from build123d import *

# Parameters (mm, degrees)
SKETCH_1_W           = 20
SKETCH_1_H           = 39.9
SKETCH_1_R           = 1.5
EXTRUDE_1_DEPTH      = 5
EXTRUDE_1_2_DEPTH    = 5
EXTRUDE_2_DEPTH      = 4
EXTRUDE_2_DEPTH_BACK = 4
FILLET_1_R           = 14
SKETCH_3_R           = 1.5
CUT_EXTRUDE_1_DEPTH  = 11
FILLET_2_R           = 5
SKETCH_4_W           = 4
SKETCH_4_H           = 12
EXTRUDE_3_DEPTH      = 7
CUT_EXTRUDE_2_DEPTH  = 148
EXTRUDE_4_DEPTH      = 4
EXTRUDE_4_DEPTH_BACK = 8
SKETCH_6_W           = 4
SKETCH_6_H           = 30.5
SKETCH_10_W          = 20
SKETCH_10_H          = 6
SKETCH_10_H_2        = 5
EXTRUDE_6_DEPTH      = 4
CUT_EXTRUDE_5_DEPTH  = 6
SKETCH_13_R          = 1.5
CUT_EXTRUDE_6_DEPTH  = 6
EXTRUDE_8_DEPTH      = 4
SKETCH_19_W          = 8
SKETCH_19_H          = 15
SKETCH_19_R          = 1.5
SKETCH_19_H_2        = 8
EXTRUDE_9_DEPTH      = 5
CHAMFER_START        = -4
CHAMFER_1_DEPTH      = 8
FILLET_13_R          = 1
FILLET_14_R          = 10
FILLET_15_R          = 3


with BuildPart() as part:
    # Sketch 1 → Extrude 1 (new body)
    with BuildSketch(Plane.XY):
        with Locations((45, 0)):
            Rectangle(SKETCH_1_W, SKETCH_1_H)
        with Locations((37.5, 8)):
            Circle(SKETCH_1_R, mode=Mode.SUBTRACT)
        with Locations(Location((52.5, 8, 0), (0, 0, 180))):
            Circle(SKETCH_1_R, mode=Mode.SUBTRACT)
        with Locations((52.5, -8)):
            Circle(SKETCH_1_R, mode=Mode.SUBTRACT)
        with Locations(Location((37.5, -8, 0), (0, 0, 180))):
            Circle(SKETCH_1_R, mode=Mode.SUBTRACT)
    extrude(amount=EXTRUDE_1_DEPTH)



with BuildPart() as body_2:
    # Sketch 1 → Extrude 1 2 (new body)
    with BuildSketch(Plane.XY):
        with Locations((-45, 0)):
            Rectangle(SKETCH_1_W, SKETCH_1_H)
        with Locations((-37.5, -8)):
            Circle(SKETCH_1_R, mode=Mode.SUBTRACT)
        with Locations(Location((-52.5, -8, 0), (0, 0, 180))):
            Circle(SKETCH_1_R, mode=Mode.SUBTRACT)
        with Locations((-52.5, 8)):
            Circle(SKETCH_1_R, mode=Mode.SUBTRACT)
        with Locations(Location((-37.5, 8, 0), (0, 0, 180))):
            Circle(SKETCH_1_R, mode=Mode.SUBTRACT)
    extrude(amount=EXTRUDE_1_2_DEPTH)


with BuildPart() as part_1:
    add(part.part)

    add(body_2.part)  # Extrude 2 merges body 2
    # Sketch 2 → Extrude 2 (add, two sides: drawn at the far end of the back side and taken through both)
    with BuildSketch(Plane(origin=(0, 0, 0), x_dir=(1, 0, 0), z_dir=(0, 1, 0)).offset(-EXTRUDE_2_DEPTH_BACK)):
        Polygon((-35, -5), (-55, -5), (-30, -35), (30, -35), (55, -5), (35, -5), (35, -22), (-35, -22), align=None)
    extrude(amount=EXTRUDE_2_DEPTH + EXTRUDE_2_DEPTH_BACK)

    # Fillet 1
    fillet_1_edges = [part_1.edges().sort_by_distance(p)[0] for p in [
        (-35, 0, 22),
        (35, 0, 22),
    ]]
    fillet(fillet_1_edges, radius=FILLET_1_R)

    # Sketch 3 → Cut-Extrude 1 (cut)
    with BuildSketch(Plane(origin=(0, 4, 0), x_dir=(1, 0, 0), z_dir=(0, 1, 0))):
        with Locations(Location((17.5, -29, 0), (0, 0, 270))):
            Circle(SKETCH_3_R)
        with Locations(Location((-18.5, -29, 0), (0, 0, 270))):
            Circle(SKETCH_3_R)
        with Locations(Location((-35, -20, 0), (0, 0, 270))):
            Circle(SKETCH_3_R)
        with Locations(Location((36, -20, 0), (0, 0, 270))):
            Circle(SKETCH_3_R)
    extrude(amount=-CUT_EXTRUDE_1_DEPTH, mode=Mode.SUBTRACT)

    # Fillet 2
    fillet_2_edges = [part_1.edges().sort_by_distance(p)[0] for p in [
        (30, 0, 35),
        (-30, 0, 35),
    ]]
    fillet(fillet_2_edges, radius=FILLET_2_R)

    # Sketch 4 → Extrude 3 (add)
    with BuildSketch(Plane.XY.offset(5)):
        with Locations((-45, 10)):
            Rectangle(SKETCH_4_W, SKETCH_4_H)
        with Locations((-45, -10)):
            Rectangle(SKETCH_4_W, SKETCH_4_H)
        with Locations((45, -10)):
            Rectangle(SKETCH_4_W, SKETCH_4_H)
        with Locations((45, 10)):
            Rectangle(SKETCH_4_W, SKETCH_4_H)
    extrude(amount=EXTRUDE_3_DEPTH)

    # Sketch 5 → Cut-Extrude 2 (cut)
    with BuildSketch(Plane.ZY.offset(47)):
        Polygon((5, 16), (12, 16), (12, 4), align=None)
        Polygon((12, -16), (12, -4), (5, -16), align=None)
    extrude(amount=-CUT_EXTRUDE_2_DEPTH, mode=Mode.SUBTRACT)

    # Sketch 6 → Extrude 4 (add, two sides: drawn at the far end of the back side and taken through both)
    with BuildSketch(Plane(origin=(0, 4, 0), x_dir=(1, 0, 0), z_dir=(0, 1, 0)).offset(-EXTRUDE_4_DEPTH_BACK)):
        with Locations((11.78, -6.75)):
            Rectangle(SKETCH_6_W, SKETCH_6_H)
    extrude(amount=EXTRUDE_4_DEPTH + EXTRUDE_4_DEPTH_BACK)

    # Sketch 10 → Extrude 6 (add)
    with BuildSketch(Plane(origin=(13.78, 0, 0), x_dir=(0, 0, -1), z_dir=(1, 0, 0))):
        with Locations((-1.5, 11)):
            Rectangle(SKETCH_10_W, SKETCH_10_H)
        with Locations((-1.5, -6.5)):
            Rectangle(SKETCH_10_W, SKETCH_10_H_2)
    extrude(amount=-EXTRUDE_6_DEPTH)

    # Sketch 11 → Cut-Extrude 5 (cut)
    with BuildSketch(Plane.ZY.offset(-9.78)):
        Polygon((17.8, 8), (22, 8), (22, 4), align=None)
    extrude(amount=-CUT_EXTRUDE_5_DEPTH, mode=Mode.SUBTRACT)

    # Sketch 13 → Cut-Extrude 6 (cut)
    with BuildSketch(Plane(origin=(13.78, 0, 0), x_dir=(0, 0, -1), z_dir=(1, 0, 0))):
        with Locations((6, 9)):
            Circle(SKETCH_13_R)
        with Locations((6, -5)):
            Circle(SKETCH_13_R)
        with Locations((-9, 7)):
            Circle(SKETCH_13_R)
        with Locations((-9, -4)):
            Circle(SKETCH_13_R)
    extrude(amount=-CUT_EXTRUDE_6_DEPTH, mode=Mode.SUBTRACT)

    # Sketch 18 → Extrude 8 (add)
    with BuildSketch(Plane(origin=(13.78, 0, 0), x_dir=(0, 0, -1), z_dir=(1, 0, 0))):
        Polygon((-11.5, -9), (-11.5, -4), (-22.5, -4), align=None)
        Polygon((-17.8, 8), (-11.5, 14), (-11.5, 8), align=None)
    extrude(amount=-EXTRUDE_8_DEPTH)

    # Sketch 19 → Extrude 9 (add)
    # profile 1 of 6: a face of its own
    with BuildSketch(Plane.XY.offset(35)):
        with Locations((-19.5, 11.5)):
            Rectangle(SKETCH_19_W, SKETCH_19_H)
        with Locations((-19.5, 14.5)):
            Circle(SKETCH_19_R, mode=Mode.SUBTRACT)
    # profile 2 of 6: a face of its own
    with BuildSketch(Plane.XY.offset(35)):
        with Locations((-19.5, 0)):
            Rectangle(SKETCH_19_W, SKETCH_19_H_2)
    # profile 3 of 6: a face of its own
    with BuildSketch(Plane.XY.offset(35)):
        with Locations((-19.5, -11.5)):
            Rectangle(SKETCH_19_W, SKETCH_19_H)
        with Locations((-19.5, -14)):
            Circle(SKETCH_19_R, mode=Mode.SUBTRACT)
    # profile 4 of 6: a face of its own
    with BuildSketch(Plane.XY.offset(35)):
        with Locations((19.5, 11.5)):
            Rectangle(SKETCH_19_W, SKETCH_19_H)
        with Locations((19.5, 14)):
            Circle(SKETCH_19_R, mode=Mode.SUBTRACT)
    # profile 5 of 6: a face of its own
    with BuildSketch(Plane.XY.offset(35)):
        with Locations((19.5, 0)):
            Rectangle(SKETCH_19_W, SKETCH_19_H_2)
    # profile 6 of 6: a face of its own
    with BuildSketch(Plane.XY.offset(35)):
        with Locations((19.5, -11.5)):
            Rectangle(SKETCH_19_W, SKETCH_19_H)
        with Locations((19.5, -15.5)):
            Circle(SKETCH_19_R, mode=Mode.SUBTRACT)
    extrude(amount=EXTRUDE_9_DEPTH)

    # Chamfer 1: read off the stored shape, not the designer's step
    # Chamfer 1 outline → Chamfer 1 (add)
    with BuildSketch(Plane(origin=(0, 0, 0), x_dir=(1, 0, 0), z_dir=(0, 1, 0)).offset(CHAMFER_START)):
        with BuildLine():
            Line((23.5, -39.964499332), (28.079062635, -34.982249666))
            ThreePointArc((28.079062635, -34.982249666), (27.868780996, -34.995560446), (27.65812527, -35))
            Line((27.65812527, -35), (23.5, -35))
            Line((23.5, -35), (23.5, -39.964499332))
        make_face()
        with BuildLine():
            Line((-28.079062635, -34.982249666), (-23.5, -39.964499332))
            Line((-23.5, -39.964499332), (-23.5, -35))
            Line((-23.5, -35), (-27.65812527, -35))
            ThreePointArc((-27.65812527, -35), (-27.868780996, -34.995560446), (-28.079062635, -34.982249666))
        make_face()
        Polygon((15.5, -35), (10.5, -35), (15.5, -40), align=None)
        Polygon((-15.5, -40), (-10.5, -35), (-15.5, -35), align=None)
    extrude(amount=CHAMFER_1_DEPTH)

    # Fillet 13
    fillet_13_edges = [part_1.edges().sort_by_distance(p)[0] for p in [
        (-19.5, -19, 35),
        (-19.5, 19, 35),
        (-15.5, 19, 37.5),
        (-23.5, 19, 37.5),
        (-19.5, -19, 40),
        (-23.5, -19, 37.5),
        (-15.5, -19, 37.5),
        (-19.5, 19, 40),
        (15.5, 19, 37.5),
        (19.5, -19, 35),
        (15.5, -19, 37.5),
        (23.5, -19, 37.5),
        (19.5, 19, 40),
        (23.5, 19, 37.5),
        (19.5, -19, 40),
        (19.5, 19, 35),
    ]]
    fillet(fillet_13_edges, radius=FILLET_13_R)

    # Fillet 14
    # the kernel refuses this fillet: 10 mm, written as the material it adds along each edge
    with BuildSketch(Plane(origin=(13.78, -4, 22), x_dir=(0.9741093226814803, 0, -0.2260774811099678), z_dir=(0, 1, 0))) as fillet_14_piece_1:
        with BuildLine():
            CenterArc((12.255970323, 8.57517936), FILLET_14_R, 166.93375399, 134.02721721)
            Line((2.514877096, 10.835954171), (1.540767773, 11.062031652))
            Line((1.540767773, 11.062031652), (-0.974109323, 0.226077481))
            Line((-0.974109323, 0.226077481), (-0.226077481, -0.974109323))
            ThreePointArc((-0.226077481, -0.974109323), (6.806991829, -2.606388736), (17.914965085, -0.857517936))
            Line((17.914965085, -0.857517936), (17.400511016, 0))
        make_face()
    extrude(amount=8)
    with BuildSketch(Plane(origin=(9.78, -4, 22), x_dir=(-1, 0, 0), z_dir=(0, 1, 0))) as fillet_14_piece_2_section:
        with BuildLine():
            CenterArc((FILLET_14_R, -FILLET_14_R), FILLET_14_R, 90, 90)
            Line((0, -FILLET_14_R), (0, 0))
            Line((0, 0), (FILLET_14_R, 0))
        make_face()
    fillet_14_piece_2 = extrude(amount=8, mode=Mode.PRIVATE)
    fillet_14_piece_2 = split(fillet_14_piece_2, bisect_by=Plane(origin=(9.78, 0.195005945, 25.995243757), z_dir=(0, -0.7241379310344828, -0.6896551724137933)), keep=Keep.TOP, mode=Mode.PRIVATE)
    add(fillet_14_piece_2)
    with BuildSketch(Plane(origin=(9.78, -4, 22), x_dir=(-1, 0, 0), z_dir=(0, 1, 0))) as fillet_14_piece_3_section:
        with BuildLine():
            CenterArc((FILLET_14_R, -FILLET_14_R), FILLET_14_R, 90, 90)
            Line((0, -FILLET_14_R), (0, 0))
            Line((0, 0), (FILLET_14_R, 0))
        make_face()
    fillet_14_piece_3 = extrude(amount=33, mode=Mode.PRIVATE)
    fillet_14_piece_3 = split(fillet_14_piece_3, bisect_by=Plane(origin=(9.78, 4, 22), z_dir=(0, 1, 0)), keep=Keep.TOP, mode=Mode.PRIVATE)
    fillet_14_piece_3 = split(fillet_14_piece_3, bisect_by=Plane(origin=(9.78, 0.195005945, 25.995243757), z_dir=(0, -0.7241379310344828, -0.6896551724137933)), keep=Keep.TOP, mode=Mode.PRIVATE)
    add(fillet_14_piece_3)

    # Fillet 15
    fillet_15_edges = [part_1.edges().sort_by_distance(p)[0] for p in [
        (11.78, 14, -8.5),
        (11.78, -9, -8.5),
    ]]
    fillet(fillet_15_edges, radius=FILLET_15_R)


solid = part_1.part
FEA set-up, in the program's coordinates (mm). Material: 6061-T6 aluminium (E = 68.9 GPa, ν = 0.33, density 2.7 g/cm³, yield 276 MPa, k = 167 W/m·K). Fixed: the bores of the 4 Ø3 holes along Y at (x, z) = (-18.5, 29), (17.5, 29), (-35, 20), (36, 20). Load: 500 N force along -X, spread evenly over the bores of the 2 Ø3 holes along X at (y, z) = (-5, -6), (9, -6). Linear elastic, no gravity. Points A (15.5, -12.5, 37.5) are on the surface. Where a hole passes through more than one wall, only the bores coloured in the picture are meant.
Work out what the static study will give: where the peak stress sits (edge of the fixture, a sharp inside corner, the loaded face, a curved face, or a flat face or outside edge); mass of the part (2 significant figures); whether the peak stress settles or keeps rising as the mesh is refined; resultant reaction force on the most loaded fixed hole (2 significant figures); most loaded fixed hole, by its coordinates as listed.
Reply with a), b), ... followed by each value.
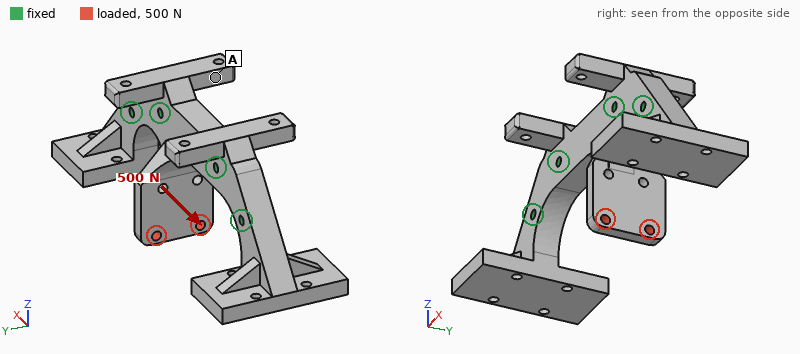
a) a sharp inside corner
b) 70 g
c) keeps rising
d) 540 N
e) (-18.5, 29)
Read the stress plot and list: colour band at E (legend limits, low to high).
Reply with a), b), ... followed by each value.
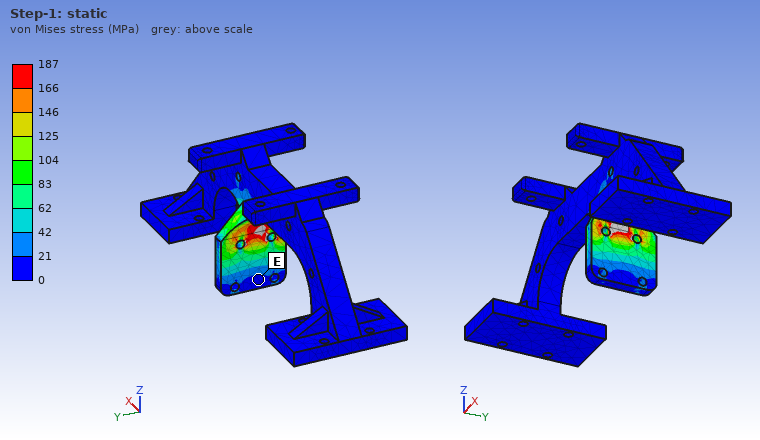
a) 0 to 21 MPa
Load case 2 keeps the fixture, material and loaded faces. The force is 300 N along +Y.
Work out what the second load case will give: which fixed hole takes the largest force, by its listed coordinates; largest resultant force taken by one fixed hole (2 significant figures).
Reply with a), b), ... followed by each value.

a) (17.5, 29)
b) 290 N
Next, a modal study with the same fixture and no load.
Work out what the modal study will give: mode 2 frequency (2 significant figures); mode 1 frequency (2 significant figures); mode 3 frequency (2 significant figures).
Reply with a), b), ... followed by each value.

a) 3900 Hz
b) 3800 Hz
c) 4400 Hz
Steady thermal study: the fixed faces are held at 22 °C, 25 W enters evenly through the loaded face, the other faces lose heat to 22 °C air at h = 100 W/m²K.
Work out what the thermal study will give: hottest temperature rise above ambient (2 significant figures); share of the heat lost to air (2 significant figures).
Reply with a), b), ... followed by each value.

a) 56 K
b) 24 %
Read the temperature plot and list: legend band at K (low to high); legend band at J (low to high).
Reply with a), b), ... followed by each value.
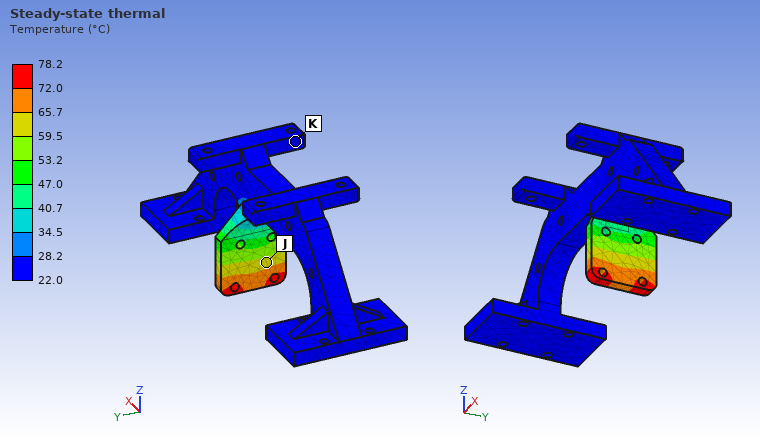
a) 22.0 to 28.2 °C
b) 59.5 to 65.7 °C
